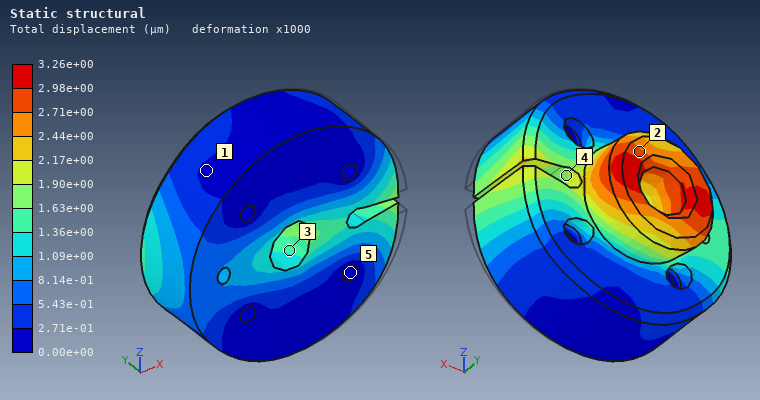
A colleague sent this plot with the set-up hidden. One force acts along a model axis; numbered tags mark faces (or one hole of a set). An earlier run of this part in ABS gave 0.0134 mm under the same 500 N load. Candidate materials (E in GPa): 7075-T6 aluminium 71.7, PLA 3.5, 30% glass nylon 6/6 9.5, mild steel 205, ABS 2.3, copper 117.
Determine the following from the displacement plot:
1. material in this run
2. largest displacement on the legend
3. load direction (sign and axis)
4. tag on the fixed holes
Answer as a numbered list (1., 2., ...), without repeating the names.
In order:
1. 30% glass nylon 6/6
2. 3.26e+00 µm
3. -X
4. 5
